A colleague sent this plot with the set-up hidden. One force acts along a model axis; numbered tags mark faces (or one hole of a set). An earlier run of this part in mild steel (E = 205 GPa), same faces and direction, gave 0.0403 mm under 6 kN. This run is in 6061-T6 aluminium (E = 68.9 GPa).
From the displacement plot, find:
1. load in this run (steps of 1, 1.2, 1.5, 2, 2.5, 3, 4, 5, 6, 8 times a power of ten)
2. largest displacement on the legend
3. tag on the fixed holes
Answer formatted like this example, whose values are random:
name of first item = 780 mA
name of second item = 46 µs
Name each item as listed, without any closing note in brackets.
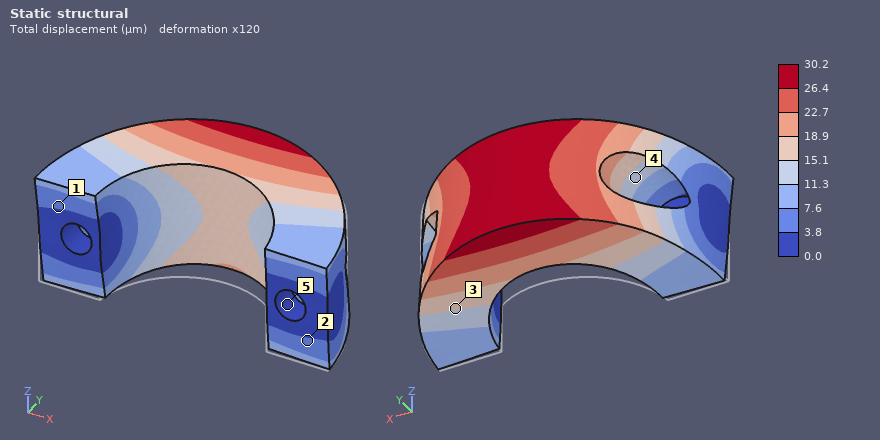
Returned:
load in this run = 1.5 kN
largest displacement on the legend = 30.2 µm
tag on the fixed holes = 5
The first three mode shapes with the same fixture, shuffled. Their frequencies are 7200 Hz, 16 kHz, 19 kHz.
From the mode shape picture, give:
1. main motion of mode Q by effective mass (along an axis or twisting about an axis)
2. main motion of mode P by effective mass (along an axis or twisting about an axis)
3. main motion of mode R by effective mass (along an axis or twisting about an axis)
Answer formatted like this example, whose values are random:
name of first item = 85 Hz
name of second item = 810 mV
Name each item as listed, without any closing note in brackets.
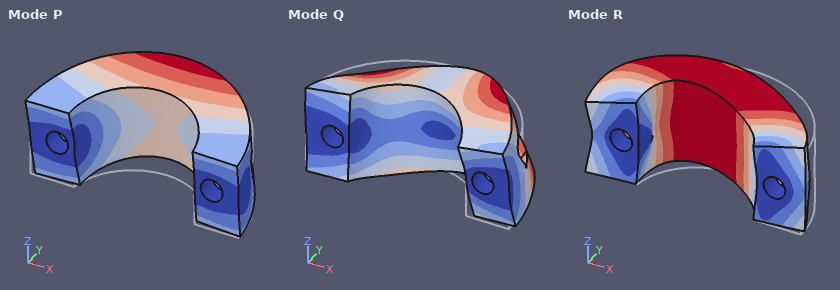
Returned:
main motion of mode Q by effective mass = twisting about Y
main motion of mode P by effective mass = along Z
main motion of mode R by effective mass = along X
